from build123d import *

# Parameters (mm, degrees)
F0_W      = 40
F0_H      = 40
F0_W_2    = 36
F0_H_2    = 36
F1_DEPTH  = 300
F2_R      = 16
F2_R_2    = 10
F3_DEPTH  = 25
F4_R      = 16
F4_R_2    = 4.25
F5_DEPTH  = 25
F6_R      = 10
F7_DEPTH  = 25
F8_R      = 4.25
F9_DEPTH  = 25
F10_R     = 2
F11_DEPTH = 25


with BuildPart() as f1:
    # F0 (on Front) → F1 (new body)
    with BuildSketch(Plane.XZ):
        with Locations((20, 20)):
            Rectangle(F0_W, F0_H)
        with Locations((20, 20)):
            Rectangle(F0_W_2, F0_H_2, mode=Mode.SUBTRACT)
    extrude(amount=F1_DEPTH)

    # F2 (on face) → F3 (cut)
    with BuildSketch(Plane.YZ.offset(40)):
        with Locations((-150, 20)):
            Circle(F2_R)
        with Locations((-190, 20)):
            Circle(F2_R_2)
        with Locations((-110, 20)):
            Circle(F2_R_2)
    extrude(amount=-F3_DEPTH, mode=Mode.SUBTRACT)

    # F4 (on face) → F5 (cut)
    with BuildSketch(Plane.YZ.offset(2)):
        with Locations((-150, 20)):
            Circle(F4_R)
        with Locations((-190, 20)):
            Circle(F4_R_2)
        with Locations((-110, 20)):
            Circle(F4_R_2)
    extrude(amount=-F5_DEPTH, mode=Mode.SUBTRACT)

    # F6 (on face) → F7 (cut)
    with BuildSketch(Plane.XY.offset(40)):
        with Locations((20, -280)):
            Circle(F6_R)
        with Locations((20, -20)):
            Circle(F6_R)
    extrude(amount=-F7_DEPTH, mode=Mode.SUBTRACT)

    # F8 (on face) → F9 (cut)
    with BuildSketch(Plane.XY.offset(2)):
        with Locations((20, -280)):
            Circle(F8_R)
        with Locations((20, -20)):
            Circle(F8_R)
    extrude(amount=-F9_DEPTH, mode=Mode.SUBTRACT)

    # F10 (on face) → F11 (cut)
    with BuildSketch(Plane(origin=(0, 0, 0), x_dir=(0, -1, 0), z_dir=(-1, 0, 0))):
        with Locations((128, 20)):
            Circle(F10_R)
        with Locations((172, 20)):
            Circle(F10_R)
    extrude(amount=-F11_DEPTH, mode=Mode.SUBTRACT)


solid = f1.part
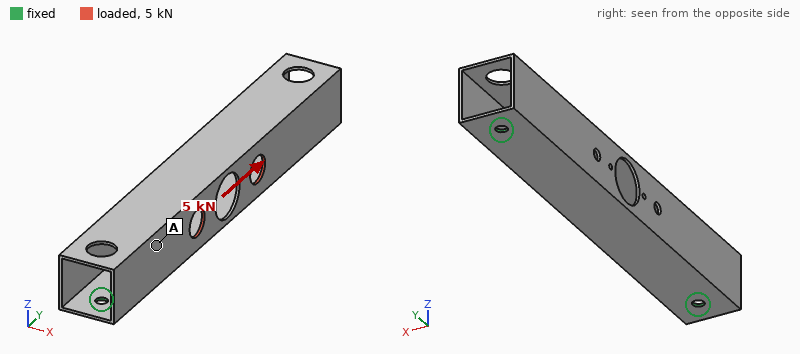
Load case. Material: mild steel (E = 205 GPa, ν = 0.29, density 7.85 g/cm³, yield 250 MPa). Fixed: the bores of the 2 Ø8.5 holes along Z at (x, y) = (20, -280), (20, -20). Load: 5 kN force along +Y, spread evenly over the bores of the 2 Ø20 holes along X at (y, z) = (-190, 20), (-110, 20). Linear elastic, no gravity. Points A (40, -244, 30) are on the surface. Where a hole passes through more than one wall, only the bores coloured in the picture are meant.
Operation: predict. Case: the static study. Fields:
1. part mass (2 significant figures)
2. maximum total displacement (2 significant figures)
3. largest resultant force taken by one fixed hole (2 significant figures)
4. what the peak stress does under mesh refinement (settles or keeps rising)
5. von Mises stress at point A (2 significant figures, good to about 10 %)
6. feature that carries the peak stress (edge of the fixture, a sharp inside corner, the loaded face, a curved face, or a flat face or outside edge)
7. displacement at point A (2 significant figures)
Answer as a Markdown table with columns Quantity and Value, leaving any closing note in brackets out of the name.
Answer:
| Quantity | Value |
|---|---|
| part mass | 670 g |
| maximum total displacement | 58 µm |
| largest resultant force taken by one fixed hole | 2.6 kN |
| what the peak stress does under mesh refinement | keeps rising |
| von Mises stress at point A | 10 MPa |
| feature that carries the peak stress | edge of the fixture |
| displacement at point A | 27 µm |
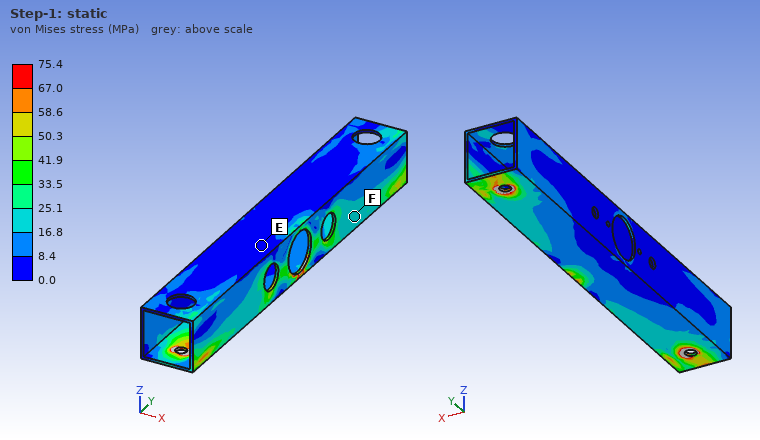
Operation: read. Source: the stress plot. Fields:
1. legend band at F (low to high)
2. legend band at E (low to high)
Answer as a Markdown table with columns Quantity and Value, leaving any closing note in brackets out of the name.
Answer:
| Quantity | Value |
|---|---|
| legend band at F | 16.8 to 25.1 MPa |
| legend band at E | 0.0 to 8.4 MPa |
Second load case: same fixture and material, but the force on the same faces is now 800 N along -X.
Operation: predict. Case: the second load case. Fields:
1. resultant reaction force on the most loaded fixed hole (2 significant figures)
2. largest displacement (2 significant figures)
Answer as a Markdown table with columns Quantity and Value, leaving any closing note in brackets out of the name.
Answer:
| Quantity | Value |
|---|---|
| resultant reaction force on the most loaded fixed hole | 400 N |
| largest displacement | 0.26 mm |
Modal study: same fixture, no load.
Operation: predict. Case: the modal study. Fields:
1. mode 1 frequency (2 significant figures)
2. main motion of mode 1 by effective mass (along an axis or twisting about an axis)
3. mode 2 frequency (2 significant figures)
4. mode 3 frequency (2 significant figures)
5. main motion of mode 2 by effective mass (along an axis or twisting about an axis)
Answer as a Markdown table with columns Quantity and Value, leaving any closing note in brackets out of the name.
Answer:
| Quantity | Value |
|---|---|
| mode 1 frequency | 360 Hz |
| main motion of mode 1 by effective mass | along X |
| mode 2 frequency | 960 Hz |
| mode 3 frequency | 1400 Hz |
| main motion of mode 2 by effective mass | along Z |
